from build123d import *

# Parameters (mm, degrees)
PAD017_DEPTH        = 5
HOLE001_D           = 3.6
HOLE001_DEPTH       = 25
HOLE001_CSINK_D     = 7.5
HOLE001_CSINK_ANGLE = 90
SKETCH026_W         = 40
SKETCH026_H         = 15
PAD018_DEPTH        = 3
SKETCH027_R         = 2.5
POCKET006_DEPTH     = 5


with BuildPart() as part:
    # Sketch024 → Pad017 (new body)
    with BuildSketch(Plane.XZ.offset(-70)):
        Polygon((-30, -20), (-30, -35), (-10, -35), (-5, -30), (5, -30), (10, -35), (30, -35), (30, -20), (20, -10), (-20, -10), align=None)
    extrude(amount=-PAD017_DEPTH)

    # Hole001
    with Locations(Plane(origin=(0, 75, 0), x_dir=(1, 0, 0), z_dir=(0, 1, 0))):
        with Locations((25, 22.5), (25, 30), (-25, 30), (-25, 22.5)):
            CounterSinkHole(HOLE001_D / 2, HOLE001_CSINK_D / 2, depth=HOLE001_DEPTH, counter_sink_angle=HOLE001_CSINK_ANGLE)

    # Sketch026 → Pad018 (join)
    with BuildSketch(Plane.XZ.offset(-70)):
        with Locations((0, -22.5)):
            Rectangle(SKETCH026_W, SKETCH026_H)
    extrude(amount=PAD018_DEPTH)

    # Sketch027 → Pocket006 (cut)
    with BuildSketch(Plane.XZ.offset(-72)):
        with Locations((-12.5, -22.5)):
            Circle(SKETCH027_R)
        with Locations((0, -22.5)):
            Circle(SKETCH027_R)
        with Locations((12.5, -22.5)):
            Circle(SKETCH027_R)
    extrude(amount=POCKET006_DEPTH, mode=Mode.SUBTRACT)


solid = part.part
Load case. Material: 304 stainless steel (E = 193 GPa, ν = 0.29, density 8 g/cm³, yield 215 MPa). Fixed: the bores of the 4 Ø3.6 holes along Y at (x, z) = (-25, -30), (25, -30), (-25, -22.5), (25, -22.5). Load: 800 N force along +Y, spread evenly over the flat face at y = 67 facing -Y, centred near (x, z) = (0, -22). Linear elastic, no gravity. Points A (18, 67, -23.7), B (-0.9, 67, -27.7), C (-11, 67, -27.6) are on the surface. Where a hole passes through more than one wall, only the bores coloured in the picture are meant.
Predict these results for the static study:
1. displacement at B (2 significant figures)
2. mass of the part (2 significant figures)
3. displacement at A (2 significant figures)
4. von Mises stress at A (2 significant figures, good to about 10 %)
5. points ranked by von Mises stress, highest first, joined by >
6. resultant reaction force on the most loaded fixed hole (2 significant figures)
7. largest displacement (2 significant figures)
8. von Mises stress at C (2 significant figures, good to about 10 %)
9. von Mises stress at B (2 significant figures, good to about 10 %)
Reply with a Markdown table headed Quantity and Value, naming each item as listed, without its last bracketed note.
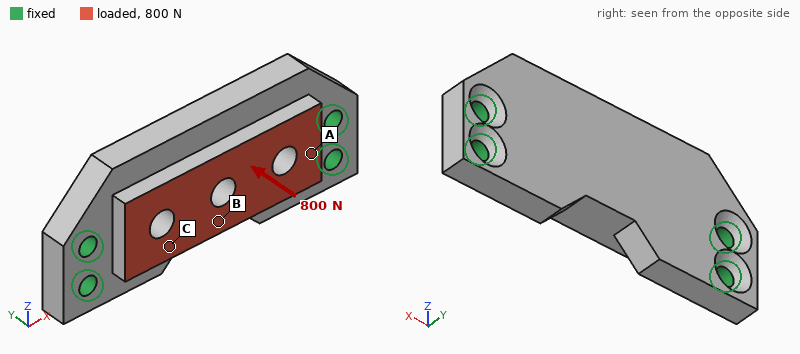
| Quantity | Value |
|---|---|
| displacement at B | 5.9 µm |
| mass of the part | 62 g |
| displacement at A | 2.8 µm |
| von Mises stress at A | 6.3 MPa |
| points ranked by von Mises stress, highest first, joined by > | B > C > A |
| resultant reaction force on the most loaded fixed hole | 330 N |
| largest displacement | 8.4 µm |
| von Mises stress at C | 14 MPa |
| von Mises stress at B | 24 MPa |
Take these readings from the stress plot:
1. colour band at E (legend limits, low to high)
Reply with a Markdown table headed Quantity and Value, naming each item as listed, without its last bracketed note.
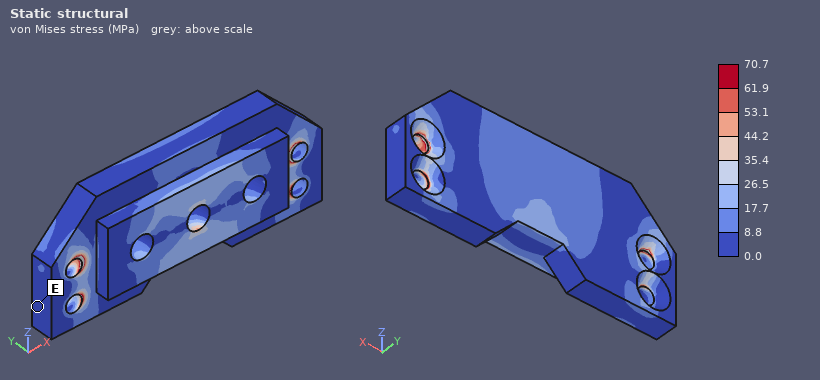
| Quantity | Value |
|---|---|
| colour band at E | 0.0 to 8.8 MPa |
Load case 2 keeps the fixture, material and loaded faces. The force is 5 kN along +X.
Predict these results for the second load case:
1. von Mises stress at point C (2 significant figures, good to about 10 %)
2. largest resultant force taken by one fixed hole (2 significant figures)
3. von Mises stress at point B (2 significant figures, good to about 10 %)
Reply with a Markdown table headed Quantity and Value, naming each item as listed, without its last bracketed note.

| Quantity | Value |
|---|---|
| von Mises stress at point C | 23 MPa |
| largest resultant force taken by one fixed hole | 1.6 kN |
| von Mises stress at point B | 18 MPa |
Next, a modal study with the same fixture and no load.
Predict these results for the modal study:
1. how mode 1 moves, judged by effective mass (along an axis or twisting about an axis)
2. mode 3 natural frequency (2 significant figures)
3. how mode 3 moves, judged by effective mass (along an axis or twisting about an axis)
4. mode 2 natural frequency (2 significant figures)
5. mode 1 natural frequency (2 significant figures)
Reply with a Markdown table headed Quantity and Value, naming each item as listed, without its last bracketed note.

| Quantity | Value |
|---|---|
| how mode 1 moves, judged by effective mass | along Y |
| mode 3 natural frequency | 19 kHz |
| how mode 3 moves, judged by effective mass | along Z |
| mode 2 natural frequency | 14 kHz |
| mode 1 natural frequency | 8300 Hz |
